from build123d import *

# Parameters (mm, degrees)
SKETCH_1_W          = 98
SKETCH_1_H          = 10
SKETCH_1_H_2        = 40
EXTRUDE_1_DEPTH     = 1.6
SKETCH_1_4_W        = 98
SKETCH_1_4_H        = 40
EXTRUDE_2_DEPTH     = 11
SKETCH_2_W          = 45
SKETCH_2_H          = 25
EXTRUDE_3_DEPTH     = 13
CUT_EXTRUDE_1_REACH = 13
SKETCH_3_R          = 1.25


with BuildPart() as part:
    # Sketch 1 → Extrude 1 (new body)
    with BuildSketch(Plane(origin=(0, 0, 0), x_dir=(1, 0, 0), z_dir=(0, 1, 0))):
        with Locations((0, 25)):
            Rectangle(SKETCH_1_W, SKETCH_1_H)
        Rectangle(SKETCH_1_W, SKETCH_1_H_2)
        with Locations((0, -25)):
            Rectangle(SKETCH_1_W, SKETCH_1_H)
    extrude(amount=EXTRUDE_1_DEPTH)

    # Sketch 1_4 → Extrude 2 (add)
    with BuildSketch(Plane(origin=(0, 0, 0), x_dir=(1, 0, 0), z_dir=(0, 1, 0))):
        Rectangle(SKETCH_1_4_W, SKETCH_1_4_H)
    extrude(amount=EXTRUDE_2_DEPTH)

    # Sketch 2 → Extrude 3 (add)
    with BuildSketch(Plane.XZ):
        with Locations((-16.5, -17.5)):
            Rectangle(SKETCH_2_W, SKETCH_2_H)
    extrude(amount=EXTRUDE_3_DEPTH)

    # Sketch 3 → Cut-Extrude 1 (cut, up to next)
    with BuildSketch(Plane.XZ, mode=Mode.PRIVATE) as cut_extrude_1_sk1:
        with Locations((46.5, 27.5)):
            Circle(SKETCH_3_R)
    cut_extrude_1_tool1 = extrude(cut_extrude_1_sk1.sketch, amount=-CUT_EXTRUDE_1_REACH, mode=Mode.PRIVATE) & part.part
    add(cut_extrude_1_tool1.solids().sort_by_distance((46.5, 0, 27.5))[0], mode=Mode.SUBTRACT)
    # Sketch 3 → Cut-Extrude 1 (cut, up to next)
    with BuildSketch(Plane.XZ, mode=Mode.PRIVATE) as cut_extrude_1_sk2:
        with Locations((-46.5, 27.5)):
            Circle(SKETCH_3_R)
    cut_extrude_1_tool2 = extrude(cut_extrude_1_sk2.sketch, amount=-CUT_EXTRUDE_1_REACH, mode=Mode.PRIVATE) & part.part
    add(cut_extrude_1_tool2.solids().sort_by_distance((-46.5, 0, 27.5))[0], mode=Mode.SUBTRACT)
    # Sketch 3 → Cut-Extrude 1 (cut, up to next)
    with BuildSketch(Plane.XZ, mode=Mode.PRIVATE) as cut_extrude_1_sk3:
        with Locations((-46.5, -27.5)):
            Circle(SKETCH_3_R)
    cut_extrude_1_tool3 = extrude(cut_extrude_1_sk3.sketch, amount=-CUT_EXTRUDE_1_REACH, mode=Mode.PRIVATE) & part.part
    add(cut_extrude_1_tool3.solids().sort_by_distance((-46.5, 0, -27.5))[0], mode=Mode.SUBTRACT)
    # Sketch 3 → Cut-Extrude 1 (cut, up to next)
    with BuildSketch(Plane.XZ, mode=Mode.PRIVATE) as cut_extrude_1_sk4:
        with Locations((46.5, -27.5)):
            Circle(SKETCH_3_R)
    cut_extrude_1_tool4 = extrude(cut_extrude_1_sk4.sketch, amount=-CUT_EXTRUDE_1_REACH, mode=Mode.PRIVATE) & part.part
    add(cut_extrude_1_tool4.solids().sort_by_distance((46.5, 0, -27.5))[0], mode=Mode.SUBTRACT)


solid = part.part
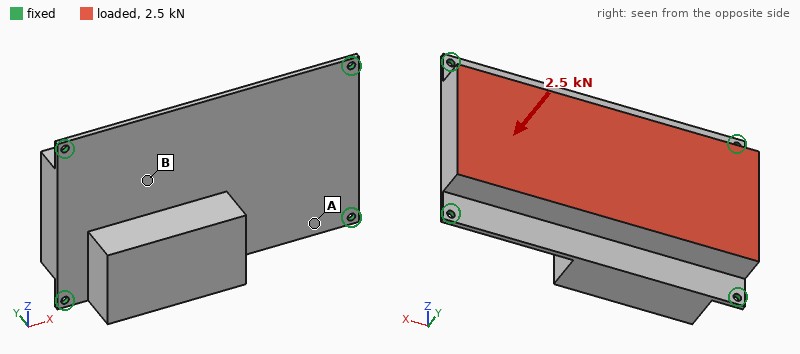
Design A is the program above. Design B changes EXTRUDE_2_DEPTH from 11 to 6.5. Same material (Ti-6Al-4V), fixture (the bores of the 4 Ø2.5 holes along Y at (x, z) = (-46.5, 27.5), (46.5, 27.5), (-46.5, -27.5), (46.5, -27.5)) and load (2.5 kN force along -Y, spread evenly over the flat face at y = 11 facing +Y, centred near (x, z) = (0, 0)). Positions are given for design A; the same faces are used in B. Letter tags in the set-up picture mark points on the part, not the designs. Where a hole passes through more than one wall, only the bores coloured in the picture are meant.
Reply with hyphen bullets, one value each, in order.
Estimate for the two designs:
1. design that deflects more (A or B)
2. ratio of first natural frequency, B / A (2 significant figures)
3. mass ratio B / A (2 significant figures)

- B
- 0.91
- 0.71
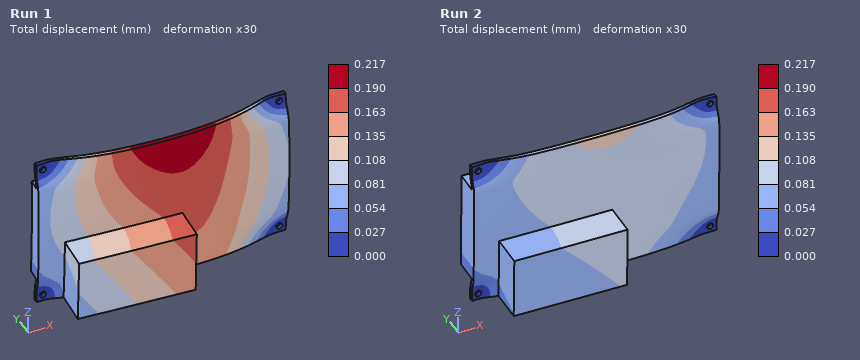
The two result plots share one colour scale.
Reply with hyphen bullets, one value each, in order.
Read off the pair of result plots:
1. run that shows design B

- Run 1
